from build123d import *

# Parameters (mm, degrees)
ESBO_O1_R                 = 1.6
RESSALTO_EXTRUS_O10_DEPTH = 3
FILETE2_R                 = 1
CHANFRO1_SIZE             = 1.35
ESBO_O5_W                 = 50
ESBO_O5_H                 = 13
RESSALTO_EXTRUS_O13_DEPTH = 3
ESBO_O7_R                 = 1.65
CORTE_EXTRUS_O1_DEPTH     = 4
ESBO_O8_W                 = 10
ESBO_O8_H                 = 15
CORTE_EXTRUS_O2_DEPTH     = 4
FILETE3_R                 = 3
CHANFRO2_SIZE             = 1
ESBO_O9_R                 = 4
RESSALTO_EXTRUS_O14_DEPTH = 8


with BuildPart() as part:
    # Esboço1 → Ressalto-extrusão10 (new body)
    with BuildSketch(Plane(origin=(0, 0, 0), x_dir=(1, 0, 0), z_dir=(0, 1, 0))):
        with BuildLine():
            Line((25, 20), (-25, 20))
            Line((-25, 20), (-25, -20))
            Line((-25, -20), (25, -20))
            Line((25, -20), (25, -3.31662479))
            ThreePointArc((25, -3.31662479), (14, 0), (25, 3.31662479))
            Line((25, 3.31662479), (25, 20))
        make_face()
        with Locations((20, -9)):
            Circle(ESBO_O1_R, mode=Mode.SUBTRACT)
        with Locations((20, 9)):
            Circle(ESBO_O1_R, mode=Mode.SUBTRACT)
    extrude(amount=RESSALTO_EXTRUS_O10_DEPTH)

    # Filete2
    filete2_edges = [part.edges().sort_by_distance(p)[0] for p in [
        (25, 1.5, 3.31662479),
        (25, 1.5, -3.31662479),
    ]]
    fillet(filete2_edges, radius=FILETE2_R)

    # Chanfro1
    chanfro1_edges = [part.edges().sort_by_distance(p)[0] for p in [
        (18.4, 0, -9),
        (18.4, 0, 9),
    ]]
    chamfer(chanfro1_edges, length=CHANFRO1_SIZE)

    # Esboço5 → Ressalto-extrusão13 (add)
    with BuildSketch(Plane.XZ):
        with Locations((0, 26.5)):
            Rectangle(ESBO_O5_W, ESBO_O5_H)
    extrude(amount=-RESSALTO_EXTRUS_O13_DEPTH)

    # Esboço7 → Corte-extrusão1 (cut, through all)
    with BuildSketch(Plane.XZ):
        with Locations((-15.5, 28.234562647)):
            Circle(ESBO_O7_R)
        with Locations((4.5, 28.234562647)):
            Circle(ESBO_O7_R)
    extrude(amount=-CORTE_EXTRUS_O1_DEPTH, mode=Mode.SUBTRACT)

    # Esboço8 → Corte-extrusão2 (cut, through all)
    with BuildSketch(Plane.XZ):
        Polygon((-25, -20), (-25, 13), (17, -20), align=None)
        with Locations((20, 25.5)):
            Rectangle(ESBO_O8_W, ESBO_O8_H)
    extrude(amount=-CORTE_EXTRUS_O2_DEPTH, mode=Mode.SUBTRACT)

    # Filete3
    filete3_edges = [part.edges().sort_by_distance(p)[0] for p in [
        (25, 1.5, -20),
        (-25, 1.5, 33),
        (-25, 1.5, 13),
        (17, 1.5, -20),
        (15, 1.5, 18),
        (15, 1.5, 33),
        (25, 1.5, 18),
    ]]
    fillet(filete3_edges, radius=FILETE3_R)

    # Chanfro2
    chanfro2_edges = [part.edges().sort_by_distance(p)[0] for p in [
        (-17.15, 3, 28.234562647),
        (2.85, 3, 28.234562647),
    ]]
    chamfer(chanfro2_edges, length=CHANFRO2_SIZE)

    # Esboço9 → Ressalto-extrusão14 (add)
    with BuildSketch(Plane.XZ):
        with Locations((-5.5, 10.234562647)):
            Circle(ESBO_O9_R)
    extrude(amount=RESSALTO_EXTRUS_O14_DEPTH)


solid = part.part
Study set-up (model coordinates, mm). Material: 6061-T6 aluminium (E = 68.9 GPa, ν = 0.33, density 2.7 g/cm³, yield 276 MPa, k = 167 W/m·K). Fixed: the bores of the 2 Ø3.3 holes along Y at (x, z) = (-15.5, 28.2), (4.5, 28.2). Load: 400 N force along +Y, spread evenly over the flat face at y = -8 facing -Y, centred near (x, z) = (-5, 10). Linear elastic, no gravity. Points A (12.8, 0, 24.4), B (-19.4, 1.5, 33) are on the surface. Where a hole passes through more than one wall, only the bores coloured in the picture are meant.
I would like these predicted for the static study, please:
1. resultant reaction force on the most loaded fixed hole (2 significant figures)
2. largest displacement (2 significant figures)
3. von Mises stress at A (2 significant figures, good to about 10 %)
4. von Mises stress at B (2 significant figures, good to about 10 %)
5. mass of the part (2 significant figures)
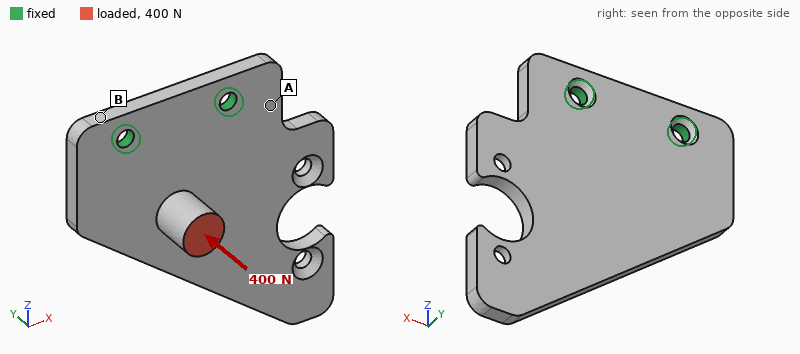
210 N
0.54 mm
69 MPa
32 MPa
14 g
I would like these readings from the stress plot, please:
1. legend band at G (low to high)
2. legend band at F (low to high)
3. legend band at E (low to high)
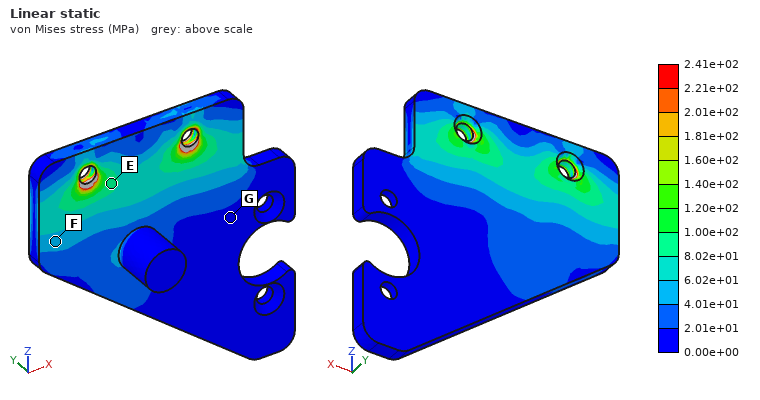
0.00e+00 to 2.01e+01 MPa
4.01e+01 to 6.02e+01 MPa
8.02e+01 to 1.00e+02 MPa
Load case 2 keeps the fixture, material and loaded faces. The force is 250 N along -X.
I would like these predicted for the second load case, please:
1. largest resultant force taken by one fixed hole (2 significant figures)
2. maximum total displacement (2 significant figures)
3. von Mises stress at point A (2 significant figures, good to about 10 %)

250 N
0.11 mm
13 MPa
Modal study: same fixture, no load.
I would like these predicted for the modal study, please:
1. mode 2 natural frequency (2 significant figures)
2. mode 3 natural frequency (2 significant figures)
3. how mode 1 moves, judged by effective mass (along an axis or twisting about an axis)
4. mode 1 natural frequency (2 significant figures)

3800 Hz
5100 Hz
along Y
1300 Hz
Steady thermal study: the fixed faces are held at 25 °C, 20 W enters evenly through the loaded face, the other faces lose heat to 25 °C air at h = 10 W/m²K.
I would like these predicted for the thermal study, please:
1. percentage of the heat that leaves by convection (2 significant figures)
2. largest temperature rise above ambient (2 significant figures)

3.0 %
45 K
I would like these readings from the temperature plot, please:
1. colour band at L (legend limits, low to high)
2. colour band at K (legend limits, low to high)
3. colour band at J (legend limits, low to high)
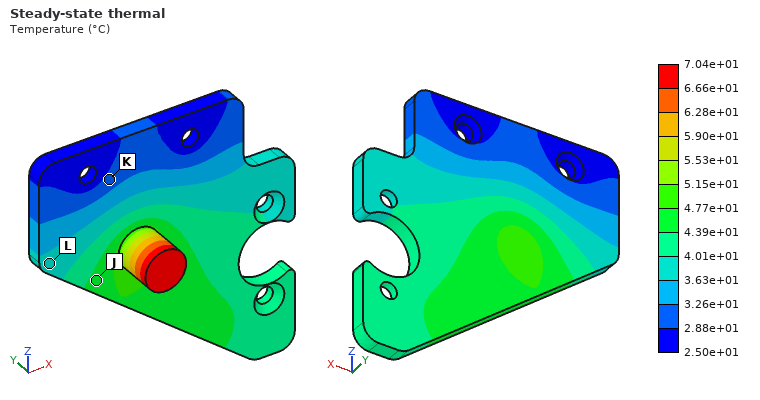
3.63e+01 to 4.01e+01 °C
2.88e+01 to 3.26e+01 °C
4.39e+01 to 4.77e+01 °C
